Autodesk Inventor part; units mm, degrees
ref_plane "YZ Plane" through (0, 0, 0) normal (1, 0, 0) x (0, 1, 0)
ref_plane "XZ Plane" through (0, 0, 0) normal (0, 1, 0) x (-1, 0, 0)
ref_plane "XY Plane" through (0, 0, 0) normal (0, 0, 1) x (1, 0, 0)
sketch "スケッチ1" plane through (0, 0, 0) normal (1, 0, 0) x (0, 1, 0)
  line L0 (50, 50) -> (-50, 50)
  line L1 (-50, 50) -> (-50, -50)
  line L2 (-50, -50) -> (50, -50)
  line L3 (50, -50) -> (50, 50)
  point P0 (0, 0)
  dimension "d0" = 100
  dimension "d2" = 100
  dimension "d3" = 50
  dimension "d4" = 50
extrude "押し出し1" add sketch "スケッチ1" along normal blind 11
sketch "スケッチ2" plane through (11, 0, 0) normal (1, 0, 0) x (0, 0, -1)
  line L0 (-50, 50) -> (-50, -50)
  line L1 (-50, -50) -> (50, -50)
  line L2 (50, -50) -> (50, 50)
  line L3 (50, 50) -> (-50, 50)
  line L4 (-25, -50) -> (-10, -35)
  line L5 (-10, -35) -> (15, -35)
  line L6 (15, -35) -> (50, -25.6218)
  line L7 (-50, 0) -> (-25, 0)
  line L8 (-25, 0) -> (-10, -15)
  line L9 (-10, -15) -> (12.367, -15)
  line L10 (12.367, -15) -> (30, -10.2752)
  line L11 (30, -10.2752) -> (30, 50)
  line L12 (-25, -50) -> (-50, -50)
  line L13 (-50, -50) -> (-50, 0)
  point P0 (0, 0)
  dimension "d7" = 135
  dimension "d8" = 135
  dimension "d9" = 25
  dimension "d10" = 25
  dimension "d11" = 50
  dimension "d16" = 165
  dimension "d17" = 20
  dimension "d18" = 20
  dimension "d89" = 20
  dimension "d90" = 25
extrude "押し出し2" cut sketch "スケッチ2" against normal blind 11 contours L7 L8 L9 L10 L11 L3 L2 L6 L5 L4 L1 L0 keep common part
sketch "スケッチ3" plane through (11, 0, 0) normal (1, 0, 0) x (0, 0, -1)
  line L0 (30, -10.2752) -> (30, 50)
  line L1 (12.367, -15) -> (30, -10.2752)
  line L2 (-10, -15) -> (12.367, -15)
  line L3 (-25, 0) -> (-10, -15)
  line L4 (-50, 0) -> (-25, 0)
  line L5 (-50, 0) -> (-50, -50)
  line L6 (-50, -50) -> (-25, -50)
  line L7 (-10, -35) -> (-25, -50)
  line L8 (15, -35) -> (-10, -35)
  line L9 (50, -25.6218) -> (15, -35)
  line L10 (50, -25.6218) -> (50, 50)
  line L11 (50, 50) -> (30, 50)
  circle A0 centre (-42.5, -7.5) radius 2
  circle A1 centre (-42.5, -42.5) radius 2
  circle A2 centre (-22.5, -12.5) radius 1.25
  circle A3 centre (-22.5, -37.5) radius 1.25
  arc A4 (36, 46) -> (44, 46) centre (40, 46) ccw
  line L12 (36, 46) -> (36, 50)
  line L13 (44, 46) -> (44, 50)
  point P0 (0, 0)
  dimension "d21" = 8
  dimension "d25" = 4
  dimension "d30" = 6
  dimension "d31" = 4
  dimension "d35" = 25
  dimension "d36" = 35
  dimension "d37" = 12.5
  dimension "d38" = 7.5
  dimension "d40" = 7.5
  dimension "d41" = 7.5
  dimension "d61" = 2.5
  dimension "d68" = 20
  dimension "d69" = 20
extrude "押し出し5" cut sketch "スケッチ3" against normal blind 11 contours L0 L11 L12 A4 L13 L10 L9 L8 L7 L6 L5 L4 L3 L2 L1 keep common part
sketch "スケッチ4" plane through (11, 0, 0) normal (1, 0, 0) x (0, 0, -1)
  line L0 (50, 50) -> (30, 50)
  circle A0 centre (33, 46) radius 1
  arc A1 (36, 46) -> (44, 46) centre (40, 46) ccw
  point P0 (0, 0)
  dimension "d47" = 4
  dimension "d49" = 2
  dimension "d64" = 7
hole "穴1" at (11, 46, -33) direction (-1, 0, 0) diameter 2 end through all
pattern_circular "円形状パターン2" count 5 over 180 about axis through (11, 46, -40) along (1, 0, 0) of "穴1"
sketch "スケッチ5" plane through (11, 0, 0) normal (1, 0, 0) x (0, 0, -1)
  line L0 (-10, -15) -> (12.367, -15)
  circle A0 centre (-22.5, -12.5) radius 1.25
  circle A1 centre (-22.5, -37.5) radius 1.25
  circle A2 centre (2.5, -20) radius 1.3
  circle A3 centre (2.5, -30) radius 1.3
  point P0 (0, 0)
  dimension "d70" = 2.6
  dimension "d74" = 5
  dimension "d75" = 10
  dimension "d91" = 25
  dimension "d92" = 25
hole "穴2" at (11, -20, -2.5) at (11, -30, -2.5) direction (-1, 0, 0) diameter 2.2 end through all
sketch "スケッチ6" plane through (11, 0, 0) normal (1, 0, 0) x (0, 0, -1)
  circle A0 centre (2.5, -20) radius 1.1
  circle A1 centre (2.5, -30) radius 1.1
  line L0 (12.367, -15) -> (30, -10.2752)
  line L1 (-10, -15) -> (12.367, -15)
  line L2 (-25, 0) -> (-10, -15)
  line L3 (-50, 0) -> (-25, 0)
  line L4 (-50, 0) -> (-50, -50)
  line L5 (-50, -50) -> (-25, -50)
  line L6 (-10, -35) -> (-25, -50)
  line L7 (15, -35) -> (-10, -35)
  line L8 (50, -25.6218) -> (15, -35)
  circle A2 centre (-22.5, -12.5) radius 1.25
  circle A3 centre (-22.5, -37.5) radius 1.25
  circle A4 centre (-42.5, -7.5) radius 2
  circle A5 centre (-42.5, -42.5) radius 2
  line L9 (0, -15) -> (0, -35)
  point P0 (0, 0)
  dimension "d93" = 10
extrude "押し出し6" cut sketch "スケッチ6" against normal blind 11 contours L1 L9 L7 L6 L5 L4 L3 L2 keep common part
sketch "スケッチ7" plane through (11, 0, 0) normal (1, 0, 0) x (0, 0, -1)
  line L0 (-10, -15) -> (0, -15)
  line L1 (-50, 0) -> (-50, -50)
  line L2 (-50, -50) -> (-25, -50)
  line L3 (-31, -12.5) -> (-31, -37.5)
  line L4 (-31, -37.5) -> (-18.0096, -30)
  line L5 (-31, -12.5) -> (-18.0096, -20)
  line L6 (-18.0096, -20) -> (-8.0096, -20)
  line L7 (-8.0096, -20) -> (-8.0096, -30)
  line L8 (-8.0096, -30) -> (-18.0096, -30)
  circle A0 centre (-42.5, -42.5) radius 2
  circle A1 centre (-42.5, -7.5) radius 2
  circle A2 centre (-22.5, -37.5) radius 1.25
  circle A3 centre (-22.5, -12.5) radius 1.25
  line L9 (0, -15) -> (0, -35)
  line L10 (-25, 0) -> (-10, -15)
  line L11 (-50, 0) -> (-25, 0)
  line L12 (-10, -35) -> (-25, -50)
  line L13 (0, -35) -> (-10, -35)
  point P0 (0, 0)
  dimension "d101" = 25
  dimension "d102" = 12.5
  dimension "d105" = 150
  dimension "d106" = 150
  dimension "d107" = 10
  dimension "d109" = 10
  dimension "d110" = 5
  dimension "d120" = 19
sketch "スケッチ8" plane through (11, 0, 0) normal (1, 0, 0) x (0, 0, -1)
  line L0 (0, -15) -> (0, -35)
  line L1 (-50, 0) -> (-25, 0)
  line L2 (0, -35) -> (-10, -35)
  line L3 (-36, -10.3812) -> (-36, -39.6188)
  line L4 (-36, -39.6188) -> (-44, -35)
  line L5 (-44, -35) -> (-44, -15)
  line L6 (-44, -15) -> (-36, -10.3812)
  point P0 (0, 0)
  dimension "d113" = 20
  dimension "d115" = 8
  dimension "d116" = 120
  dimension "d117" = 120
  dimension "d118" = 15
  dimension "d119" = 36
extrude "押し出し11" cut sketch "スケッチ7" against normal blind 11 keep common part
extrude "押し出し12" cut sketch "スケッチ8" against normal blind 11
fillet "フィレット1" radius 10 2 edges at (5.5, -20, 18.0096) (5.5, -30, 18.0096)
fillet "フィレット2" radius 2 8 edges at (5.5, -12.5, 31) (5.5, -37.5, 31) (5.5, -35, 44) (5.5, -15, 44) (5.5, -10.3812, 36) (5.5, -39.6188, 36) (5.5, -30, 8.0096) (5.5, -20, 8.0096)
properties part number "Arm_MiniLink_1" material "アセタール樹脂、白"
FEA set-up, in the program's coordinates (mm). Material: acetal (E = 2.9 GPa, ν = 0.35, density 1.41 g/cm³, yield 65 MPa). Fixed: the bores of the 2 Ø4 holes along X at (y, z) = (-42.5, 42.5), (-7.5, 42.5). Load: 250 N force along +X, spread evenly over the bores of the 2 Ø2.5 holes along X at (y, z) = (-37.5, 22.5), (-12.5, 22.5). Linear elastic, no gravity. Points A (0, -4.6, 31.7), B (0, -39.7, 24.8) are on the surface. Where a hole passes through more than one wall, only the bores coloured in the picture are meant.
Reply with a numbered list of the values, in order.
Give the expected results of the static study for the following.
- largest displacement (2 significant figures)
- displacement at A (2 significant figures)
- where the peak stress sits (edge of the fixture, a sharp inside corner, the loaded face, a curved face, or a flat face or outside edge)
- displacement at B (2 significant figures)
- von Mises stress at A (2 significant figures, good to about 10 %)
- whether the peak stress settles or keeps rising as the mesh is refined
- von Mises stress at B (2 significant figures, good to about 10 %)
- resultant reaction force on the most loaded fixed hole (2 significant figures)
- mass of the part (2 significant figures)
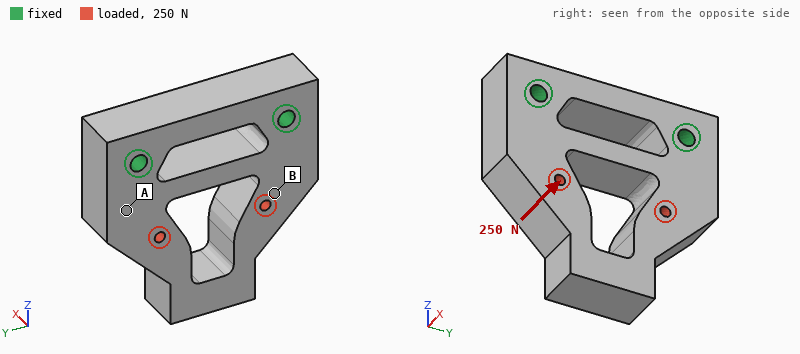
1. 0.27 mm
2. 0.046 mm
3. edge of the fixture
4. 0.099 mm
5. 4.5 MPa
6. keeps rising
7. 2.0 MPa
8. 130 N
9. 22 g
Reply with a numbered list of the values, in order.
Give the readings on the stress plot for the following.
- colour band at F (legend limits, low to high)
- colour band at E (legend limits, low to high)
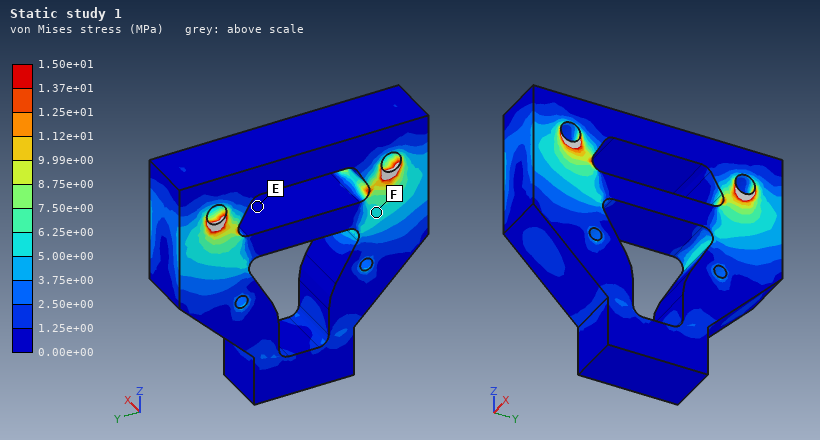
1. 5.00e+00 to 6.25e+00 MPa
2. 0.00e+00 to 1.25e+00 MPa
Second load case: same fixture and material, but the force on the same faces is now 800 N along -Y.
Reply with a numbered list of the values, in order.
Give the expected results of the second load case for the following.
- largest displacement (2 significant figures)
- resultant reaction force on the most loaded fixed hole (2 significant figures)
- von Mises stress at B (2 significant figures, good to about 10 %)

1. 0.31 mm
2. 470 N
3. 7.2 MPa
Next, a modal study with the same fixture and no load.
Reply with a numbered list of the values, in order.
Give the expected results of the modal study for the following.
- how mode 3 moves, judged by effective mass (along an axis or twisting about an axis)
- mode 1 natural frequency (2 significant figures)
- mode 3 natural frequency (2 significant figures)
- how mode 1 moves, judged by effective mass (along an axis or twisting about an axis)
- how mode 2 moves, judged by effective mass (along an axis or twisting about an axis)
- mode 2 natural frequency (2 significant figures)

1. twisting about Z
2. 1400 Hz
3. 3800 Hz
4. along X
5. along Y
6. 2500 Hz
